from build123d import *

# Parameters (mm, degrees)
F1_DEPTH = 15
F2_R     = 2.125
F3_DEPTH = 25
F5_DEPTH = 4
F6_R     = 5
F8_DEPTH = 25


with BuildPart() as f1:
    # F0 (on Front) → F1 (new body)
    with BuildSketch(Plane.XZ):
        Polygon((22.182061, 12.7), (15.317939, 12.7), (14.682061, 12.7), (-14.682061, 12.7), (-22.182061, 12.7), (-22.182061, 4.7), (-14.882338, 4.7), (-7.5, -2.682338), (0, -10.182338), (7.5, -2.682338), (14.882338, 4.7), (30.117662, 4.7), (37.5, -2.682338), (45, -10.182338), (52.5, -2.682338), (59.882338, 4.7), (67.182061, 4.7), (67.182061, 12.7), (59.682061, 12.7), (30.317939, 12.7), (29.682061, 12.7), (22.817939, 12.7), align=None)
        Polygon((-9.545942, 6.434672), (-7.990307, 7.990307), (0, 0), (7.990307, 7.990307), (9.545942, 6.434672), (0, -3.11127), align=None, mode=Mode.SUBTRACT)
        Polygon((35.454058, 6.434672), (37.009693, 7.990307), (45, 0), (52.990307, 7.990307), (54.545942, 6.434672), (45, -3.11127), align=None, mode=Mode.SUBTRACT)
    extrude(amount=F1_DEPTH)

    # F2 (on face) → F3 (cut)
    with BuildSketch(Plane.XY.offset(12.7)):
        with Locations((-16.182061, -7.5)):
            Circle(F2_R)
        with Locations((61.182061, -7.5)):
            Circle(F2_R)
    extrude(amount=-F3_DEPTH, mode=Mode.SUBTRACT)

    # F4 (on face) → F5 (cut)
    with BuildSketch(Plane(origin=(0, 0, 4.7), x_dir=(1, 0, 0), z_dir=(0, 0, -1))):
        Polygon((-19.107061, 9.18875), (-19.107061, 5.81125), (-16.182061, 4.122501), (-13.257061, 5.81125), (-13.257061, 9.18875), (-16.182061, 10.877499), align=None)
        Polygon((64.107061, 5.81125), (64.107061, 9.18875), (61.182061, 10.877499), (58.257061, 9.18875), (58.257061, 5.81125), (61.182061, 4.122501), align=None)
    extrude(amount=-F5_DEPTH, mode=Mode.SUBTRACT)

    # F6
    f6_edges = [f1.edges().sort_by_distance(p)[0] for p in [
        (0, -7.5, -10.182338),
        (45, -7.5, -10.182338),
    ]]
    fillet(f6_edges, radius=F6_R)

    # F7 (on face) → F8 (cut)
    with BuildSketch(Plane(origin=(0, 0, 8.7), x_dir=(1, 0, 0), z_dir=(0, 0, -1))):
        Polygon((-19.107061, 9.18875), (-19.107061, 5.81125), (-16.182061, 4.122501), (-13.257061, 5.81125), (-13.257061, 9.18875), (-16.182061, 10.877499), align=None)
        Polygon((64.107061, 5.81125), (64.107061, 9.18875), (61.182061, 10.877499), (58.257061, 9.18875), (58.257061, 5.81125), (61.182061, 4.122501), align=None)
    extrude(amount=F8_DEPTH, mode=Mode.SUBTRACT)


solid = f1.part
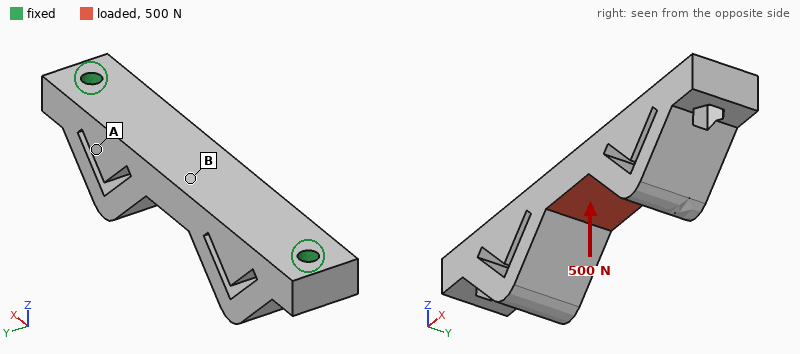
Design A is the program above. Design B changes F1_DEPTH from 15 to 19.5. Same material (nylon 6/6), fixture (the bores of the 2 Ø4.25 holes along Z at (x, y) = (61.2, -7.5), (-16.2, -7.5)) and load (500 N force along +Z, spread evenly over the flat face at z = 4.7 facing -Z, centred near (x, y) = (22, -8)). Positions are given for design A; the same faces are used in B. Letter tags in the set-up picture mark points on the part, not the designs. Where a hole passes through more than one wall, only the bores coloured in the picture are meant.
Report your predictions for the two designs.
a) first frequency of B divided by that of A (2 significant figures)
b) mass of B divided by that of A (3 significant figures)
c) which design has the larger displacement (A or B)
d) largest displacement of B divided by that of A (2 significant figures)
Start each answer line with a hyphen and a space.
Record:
- 0.95
- 1.31
- A
- 0.87
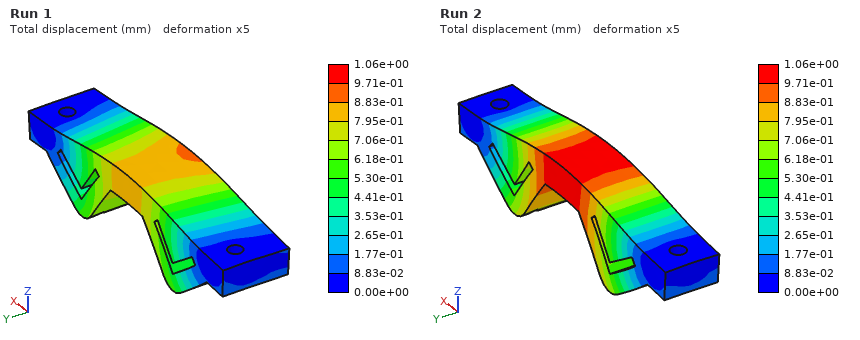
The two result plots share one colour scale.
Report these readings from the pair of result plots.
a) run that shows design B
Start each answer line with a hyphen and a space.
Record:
- Run 1
